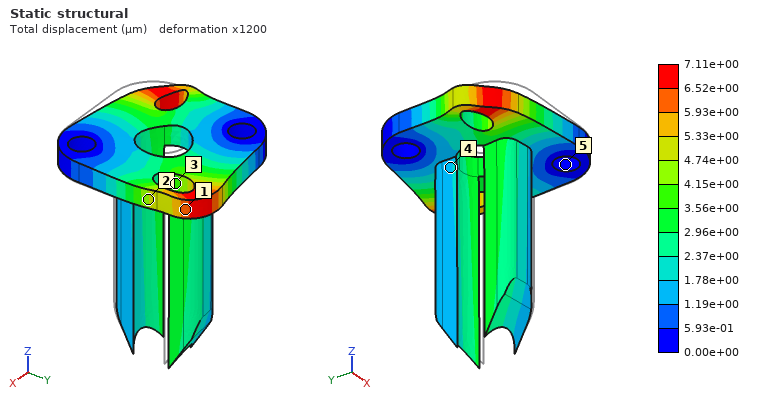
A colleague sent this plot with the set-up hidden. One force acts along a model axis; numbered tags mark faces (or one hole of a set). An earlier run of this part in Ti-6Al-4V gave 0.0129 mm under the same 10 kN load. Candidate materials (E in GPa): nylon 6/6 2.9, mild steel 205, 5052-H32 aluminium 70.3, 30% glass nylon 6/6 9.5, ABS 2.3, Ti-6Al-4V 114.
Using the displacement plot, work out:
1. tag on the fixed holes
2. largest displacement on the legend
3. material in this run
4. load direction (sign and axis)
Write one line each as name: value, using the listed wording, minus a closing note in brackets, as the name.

tag on the fixed holes: 5
largest displacement on the legend: 7.11e+00 µm
material in this run: mild steel
load direction: +Y
